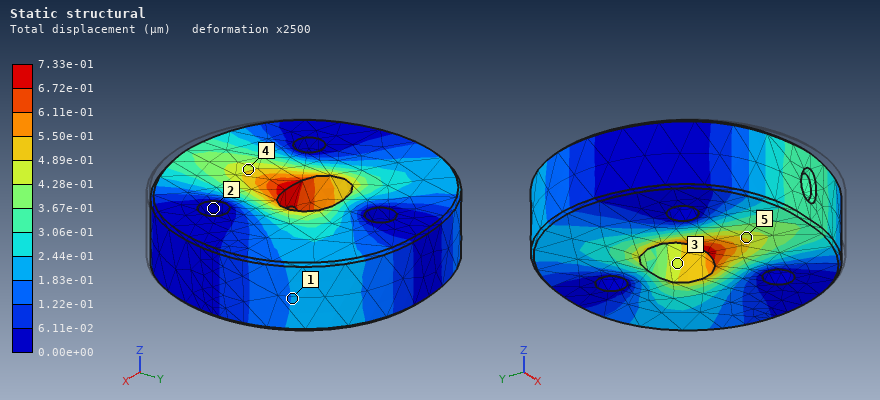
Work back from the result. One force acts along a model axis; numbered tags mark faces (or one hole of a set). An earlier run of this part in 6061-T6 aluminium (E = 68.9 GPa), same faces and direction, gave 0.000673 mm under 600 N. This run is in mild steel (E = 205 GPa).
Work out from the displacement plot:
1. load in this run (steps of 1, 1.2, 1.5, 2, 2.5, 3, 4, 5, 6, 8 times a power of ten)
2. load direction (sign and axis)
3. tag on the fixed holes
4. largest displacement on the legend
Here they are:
2 kN
+Y
2
7.33e-01 µm
